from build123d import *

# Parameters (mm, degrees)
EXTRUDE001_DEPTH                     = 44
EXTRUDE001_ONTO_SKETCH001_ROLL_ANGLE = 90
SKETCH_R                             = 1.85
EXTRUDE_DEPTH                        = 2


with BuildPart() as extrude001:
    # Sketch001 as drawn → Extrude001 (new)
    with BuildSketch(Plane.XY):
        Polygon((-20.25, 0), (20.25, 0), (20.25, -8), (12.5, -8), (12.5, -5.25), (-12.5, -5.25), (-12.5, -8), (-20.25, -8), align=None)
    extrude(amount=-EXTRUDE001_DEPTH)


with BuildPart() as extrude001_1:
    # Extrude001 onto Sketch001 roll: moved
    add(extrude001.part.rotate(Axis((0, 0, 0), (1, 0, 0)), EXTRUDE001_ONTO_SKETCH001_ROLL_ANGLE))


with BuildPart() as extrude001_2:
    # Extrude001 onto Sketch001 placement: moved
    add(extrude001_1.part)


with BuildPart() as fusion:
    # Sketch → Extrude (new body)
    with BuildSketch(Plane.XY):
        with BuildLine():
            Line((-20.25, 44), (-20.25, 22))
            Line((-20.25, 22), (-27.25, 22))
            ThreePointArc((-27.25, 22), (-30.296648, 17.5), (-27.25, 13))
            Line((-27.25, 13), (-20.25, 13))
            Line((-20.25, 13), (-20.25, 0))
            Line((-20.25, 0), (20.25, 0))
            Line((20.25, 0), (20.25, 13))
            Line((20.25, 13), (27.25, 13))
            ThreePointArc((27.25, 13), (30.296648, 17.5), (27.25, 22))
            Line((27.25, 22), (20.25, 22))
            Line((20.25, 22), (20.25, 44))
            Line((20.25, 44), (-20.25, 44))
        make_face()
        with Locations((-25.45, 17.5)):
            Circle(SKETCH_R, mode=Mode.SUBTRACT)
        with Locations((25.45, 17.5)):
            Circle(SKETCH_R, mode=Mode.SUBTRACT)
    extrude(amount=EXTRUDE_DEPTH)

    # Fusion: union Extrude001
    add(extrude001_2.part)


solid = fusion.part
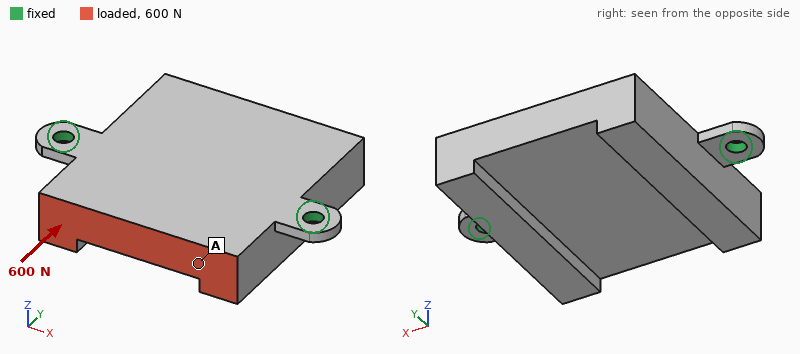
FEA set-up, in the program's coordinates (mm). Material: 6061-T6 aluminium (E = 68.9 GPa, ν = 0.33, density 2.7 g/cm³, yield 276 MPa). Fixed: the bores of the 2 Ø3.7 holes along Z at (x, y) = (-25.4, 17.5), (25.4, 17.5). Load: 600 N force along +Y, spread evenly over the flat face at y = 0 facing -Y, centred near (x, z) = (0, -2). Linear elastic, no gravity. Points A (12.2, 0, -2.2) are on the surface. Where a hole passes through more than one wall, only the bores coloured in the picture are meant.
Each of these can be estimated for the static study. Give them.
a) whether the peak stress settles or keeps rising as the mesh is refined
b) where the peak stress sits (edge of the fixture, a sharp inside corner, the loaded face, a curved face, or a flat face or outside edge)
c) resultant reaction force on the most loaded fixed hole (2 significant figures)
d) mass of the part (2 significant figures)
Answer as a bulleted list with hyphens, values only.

- keeps rising
- edge of the fixture
- 300 N
- 41 g
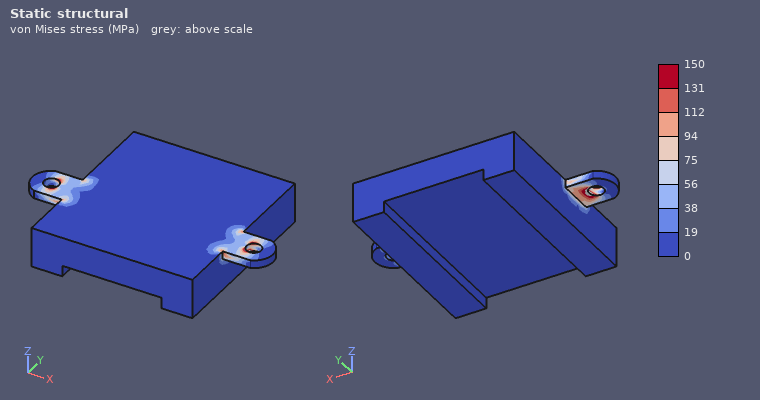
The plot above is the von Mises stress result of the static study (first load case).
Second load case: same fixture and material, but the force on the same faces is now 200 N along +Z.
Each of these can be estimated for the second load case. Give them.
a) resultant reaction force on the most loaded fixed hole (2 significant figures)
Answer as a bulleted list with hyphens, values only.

- 140 N
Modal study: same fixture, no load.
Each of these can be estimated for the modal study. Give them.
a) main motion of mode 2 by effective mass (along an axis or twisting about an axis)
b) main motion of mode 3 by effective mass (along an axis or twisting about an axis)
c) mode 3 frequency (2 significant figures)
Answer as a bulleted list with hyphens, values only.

- along Z
- twisting about Y
- 8200 Hz
